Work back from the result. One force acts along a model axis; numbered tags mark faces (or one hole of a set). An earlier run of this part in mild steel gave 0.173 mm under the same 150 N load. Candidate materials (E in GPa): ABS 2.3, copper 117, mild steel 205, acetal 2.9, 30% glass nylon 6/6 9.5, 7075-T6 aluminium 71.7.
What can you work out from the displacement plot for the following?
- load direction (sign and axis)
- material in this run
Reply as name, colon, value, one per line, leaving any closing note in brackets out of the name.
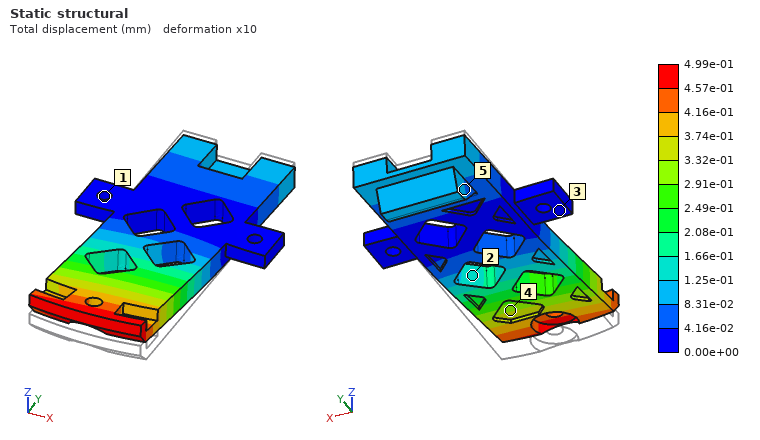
load direction: +Z
material in this run: 7075-T6 aluminium
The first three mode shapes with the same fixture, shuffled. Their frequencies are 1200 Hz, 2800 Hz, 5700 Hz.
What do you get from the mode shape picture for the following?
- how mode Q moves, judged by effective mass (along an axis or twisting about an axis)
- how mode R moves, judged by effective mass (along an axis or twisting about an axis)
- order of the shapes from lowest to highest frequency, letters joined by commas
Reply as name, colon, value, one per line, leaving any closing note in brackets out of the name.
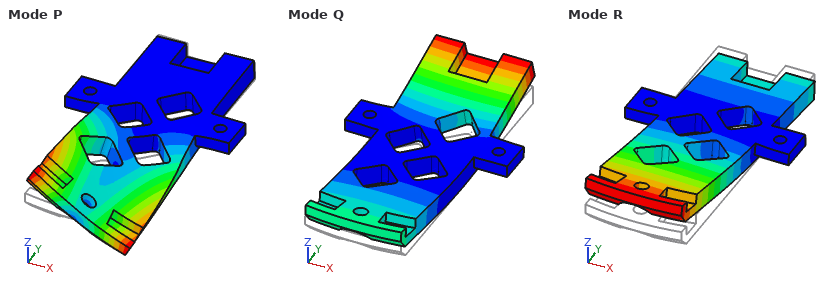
how mode Q moves, judged by effective mass: along Z
how mode R moves, judged by effective mass: along Z
order of the shapes from lowest to highest frequency, letters joined by commas: R, Q, P
